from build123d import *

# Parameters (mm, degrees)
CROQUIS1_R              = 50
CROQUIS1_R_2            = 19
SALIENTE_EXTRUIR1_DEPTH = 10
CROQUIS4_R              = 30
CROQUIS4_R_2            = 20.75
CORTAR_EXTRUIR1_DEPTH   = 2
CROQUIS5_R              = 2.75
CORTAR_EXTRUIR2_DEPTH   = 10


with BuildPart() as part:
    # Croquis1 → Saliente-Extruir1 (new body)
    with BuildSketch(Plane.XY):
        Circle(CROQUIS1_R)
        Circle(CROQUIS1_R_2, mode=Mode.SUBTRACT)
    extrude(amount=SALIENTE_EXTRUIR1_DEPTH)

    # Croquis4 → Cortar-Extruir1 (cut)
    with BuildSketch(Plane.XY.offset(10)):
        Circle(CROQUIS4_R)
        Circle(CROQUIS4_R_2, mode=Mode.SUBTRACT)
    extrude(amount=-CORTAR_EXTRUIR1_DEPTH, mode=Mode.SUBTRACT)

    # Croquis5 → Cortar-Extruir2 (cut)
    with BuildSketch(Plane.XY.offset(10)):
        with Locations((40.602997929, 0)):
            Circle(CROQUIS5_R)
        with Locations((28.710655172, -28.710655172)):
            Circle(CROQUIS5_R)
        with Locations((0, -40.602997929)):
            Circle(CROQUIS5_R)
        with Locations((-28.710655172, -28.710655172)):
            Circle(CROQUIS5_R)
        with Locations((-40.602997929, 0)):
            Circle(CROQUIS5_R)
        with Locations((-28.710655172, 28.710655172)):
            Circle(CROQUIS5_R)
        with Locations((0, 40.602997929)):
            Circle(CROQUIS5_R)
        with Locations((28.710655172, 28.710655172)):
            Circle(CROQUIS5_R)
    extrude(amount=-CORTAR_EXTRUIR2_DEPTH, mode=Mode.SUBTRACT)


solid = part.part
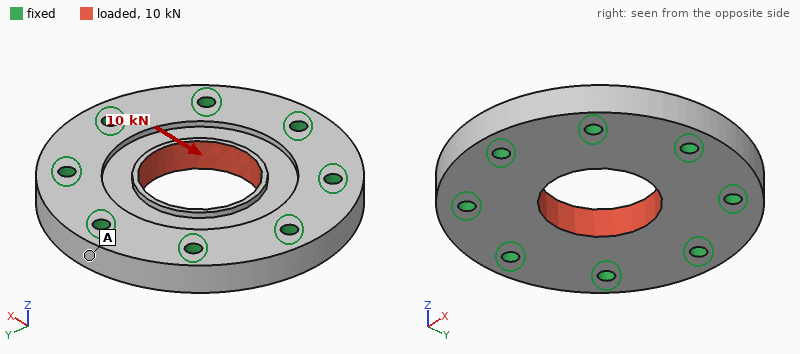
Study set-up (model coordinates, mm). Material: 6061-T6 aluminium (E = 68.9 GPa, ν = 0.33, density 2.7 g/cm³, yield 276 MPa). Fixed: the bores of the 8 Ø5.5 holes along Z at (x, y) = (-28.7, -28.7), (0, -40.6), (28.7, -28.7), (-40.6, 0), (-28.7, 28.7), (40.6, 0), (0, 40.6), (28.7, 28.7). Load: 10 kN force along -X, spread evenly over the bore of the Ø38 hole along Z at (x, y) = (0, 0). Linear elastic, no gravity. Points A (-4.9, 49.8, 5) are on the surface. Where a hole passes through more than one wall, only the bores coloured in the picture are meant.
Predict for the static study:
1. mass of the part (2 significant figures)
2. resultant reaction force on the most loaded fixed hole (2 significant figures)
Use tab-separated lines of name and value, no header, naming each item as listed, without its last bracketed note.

mass of the part	170 g
resultant reaction force on the most loaded fixed hole	1.9 kN
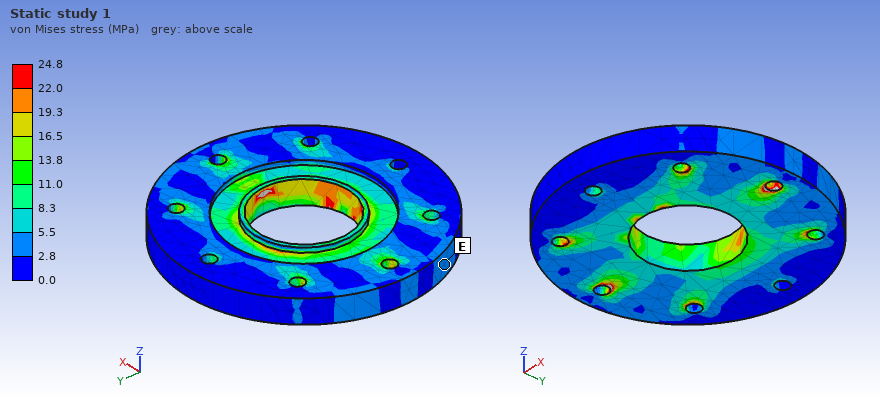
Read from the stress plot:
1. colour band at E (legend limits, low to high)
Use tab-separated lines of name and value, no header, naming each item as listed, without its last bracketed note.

colour band at E	2.8 to 5.5 MPa
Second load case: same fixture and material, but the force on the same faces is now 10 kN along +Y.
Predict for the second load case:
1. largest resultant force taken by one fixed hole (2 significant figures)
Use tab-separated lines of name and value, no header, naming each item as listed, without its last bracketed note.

largest resultant force taken by one fixed hole	1.9 kN
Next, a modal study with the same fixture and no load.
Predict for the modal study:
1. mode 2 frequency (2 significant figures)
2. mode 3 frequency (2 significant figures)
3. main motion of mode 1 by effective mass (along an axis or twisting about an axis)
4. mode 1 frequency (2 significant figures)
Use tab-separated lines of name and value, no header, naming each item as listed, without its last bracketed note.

mode 2 frequency	21 kHz
mode 3 frequency	21 kHz
main motion of mode 1 by effective mass	along Z
mode 1 frequency	17 kHz
